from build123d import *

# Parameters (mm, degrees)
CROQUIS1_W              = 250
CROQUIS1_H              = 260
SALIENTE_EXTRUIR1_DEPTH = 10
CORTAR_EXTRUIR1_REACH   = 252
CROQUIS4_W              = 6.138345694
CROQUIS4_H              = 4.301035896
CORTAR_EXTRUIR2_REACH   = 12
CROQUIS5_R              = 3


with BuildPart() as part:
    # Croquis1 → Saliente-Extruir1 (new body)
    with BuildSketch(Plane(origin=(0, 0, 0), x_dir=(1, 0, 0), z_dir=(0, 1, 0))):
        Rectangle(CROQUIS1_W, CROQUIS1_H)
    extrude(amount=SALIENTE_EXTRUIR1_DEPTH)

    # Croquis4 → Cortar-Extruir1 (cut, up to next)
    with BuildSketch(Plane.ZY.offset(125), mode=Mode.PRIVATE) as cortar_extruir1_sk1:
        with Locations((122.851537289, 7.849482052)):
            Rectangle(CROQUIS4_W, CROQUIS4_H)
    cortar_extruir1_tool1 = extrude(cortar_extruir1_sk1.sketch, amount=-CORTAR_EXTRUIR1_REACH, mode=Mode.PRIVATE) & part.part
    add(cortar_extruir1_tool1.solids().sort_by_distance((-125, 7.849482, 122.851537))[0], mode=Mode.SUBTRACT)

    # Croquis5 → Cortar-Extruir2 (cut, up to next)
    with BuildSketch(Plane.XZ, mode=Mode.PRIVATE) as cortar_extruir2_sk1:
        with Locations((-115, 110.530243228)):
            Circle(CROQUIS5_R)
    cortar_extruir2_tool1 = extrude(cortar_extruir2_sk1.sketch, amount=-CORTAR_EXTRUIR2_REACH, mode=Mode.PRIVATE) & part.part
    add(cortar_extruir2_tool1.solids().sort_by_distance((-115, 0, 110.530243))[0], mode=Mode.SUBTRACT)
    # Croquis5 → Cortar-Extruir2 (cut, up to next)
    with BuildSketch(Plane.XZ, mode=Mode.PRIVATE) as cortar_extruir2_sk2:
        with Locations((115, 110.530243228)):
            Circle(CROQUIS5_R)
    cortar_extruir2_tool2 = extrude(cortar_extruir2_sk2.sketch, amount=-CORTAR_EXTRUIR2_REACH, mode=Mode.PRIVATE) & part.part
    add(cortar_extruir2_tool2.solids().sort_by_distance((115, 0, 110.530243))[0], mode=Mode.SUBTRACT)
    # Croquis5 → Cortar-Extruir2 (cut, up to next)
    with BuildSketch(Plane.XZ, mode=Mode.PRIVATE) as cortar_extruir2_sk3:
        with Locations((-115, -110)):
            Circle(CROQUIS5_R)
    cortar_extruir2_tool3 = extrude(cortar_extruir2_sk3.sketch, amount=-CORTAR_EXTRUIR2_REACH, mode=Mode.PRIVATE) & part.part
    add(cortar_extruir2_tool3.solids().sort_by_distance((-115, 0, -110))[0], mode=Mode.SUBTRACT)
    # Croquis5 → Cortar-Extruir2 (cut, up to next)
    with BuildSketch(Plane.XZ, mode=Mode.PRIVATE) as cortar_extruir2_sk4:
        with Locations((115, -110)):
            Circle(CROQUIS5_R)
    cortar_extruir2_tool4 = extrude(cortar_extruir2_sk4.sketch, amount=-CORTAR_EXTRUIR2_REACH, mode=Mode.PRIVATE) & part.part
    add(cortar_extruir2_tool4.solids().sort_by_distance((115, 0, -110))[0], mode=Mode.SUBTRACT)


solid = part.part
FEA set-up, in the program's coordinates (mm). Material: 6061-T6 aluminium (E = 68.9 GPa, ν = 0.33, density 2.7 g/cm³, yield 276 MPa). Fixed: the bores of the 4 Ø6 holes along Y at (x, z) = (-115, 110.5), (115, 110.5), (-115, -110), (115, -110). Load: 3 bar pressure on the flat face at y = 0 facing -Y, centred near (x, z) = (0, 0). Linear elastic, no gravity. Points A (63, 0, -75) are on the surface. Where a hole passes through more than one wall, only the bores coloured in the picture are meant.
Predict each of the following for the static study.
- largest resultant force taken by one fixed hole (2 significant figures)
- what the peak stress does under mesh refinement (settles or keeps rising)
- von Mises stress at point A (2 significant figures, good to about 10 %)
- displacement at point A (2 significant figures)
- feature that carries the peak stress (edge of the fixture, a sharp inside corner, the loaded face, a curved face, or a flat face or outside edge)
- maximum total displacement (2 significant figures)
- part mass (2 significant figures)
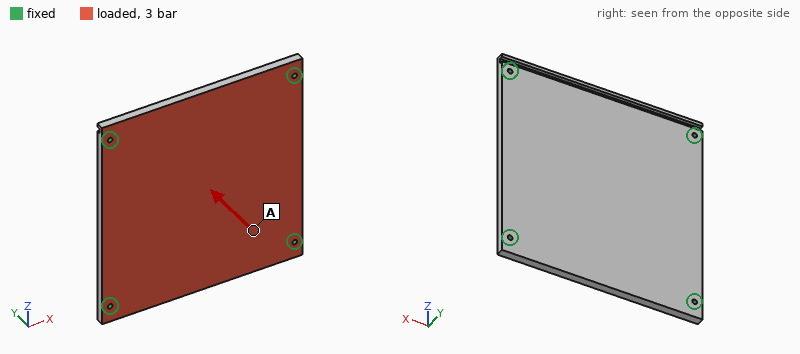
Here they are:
4.9 kN
keeps rising
28 MPa
0.64 mm
edge of the fixture
1.2 mm
1.7 kg
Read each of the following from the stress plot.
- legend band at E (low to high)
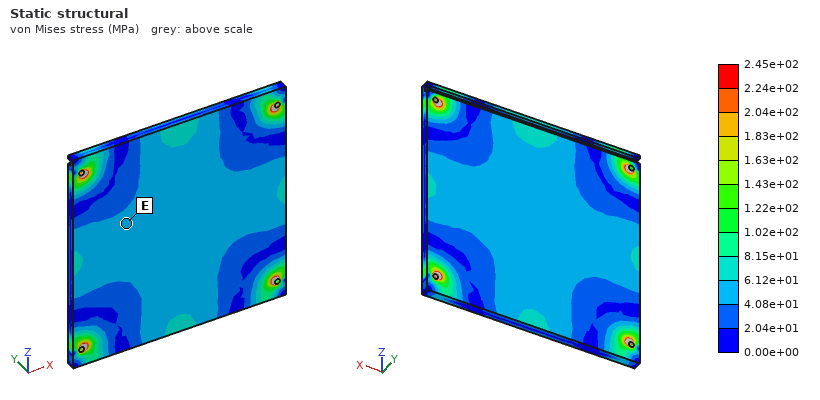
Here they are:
4.08e+01 to 6.12e+01 MPa
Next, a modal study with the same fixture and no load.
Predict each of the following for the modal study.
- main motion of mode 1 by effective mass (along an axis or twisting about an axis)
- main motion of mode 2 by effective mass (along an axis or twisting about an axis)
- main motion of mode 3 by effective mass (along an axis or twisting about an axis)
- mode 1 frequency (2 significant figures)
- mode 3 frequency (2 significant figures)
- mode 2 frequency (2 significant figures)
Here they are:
along Y
twisting about X
twisting about Z
580 Hz
1100 Hz
1000 Hz
